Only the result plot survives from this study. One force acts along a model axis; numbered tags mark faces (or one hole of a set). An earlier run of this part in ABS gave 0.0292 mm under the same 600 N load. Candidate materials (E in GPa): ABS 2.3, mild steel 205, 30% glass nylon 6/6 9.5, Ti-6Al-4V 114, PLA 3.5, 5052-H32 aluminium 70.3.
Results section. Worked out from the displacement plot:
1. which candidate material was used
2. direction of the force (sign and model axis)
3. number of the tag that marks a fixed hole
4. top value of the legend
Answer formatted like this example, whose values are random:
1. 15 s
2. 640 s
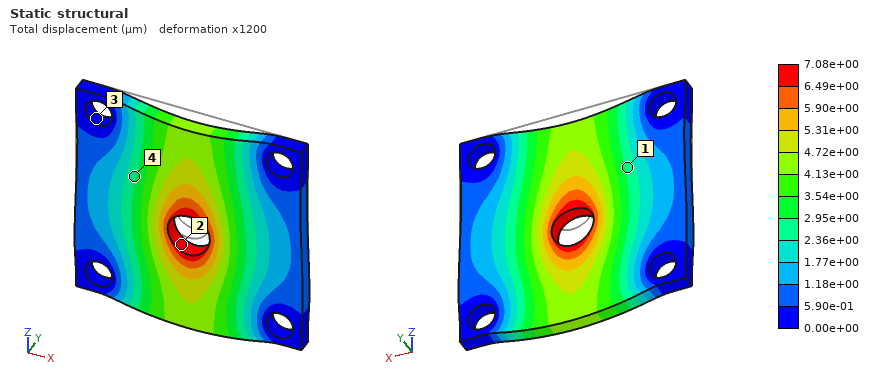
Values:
1. 30% glass nylon 6/6
2. -Z
3. 3
4. 7.08e+00 µm
